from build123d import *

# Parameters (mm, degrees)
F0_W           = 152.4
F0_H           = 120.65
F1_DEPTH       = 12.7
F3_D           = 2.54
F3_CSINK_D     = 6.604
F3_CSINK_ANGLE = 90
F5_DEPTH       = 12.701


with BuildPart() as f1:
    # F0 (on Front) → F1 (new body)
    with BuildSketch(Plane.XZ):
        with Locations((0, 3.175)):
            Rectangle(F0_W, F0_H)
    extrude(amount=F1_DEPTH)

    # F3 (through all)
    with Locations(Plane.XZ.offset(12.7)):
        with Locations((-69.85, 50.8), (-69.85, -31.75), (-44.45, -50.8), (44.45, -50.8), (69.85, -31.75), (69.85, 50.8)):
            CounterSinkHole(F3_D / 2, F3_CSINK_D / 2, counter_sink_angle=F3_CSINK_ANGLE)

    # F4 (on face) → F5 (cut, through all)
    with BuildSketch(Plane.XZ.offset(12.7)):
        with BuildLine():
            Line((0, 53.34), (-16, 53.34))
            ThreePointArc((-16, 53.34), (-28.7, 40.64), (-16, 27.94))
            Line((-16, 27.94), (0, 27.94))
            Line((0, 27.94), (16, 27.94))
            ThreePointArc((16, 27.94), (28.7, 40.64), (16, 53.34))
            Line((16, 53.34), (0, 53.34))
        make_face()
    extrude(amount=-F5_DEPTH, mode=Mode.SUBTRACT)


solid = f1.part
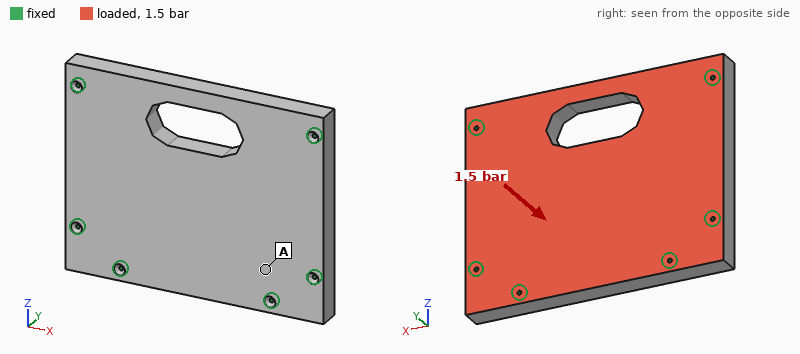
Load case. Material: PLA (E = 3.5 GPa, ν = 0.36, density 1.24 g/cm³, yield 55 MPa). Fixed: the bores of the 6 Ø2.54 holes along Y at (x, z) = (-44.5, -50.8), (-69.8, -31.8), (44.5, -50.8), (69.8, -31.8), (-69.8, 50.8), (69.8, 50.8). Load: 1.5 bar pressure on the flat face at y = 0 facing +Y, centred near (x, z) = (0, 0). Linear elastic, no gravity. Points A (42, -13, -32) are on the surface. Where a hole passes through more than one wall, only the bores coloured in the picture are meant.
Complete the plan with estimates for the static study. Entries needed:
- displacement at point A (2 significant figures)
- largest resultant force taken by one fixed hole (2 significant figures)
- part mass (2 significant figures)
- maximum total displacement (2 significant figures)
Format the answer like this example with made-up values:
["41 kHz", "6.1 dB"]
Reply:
["0.11 mm", "550 N", "270 g", "0.52 mm"]
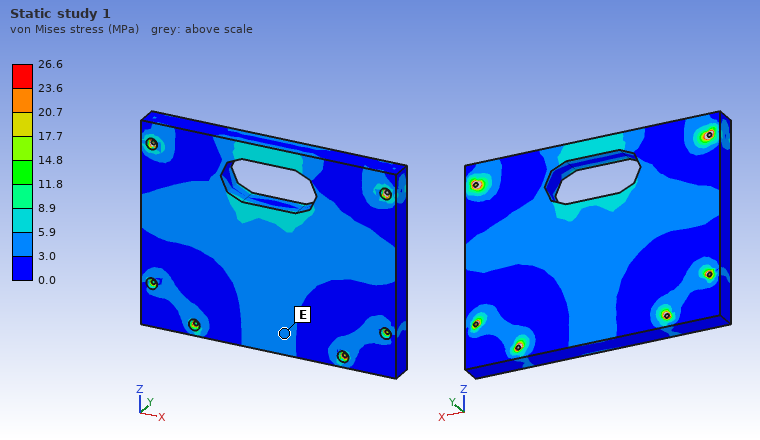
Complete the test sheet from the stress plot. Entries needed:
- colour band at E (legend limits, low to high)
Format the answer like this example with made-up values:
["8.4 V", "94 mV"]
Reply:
["3.0 to 5.9 MPa"]
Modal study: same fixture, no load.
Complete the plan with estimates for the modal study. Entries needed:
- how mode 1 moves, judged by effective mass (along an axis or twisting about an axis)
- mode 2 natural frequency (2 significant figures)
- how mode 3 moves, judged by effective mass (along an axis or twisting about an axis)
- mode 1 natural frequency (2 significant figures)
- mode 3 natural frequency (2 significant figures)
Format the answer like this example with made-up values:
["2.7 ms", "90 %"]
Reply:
["along Y", "1500 Hz", "twisting about Z", "870 Hz", "1900 Hz"]
